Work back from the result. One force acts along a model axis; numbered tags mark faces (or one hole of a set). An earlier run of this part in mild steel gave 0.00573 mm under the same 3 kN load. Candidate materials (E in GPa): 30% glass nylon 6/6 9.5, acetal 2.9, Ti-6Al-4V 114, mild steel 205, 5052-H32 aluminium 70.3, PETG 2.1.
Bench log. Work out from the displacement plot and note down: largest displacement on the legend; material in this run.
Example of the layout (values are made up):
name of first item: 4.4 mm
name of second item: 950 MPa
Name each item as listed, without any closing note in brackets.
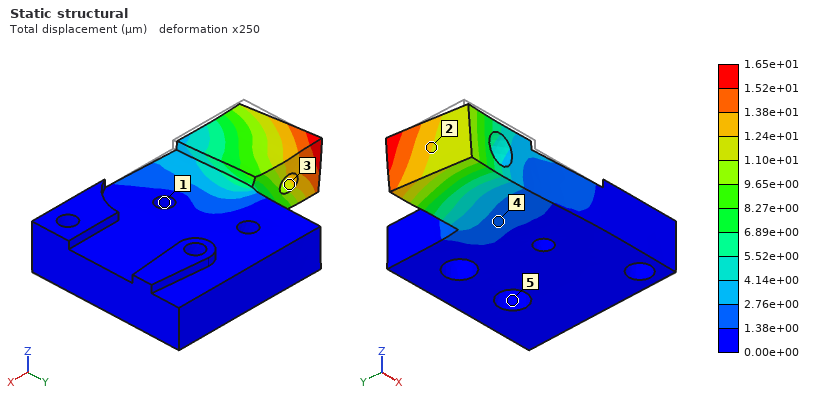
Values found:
largest displacement on the legend: 1.65e+01 µm
material in this run: 5052-H32 aluminium
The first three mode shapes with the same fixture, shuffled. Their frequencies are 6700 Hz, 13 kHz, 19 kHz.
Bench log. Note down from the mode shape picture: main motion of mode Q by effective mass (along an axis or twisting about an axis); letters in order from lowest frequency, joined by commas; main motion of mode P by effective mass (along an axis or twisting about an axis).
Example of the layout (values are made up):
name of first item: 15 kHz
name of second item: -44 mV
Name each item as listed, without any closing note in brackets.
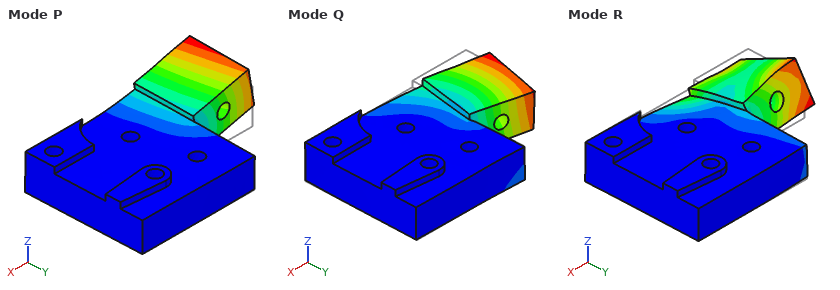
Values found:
main motion of mode Q by effective mass: along Y
letters in order from lowest frequency, joined by commas: P, Q, R
main motion of mode P by effective mass: along Z
